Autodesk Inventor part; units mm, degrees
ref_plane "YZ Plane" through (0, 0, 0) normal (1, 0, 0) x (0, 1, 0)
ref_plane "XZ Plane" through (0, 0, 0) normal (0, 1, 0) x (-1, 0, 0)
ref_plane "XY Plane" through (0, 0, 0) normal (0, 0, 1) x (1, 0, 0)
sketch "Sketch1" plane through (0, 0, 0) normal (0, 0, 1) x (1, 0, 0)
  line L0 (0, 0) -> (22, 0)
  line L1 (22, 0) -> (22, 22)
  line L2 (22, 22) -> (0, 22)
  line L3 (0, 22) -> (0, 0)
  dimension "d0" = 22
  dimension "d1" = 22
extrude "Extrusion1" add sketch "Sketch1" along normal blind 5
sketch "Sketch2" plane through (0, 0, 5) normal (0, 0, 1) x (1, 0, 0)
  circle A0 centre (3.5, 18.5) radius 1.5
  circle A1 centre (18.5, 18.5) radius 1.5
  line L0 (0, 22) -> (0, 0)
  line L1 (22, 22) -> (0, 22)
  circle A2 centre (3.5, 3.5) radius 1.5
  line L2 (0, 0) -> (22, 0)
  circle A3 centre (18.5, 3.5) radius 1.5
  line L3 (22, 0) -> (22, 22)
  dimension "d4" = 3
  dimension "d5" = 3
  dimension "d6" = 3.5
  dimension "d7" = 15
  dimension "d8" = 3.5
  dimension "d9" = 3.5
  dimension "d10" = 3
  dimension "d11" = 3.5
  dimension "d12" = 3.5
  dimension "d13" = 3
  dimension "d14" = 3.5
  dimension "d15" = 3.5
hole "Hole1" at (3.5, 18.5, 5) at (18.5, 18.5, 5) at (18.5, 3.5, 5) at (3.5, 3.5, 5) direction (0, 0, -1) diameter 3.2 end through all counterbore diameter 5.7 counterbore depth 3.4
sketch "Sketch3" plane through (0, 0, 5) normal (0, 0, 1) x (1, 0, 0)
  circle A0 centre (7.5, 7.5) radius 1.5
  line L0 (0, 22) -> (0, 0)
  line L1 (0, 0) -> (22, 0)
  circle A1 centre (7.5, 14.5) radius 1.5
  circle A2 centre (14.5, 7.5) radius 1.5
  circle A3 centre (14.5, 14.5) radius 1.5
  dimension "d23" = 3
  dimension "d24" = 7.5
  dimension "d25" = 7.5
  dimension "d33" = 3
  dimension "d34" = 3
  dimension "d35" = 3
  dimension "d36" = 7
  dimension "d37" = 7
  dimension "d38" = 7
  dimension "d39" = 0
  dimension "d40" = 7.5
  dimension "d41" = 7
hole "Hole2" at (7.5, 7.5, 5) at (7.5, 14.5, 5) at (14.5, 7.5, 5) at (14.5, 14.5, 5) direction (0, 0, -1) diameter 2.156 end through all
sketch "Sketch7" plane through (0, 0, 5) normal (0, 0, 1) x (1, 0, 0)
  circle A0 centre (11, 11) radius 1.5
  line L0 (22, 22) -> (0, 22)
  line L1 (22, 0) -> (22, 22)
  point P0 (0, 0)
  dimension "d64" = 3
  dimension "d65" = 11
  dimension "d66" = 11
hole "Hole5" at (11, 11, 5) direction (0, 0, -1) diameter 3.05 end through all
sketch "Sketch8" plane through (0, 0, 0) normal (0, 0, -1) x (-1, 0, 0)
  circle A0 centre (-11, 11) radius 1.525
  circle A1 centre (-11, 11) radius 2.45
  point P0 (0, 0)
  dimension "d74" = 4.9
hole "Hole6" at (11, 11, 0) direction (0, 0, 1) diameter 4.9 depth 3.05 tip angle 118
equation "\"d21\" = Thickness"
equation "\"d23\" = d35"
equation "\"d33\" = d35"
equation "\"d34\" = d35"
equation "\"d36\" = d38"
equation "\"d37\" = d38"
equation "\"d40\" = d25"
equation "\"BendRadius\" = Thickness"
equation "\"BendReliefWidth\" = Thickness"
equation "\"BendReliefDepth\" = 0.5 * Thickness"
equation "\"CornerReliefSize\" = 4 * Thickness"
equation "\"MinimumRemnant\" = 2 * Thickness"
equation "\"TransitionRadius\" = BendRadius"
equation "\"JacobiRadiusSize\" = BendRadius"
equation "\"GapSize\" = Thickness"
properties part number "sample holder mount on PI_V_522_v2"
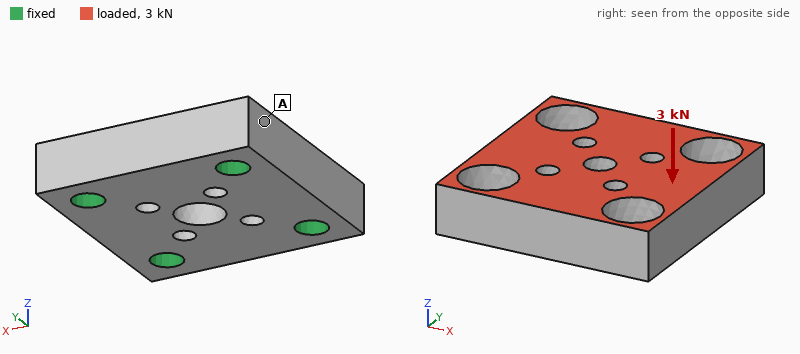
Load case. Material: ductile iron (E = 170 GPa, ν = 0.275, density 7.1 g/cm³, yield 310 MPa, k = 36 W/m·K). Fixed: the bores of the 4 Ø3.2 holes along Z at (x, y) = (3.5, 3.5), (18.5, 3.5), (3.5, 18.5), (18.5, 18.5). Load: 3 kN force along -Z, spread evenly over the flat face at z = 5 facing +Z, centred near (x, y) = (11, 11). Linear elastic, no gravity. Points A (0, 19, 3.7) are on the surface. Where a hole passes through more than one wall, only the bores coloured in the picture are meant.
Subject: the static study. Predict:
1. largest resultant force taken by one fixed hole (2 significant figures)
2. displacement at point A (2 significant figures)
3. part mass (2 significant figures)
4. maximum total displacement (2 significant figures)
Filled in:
820 N
0.77 µm
13 g
4.3 µm
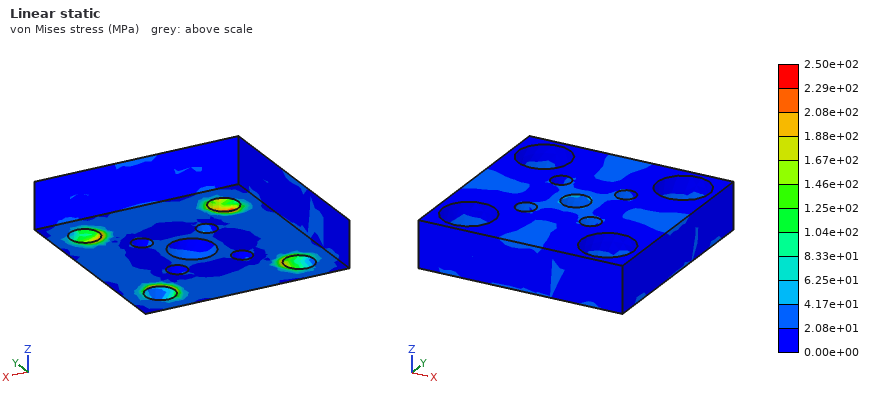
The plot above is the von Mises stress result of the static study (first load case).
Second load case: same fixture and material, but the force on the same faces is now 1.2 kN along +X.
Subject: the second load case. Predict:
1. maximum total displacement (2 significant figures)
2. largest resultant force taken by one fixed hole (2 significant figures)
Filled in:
1.8 µm
340 N
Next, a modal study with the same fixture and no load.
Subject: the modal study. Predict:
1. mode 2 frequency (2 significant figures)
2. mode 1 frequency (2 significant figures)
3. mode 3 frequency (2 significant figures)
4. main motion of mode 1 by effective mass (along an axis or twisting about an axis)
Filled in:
54 kHz
45 kHz
54 kHz
along Z
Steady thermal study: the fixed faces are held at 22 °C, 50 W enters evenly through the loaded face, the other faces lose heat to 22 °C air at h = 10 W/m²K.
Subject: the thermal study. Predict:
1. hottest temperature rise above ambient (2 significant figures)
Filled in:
65 K
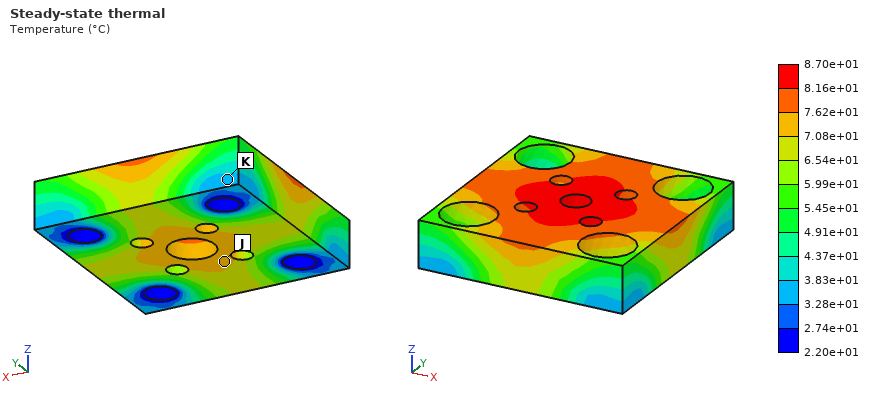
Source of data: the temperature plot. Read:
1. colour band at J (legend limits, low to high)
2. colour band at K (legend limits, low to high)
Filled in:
7.08e+01 to 7.62e+01 °C
3.28e+01 to 3.83e+01 °C
